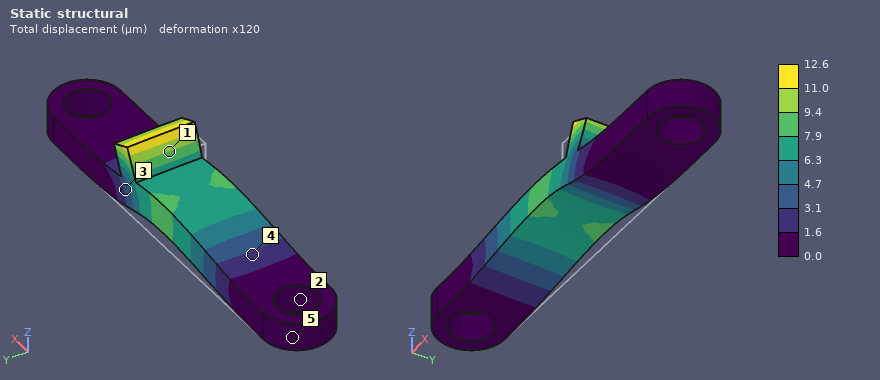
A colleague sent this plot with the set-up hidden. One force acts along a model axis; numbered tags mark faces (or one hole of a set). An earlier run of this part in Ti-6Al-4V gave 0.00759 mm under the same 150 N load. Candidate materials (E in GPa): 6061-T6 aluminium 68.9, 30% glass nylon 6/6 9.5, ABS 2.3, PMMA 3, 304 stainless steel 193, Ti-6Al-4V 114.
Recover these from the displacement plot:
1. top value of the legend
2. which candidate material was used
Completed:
12.6 µm
6061-T6 aluminium
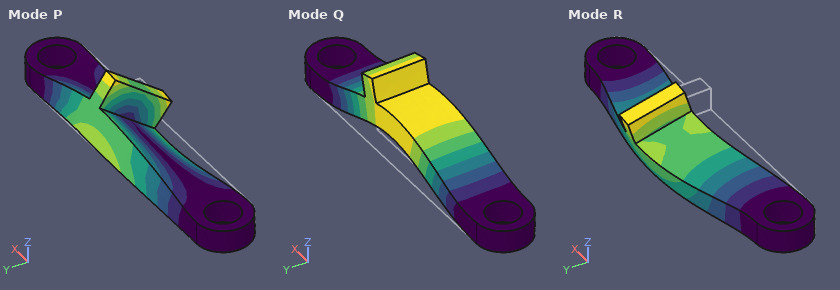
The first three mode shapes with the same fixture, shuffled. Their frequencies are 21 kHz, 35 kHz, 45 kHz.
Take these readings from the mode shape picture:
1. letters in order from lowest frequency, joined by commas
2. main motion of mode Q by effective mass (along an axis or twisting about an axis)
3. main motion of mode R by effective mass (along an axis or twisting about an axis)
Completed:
Q, R, P
along Z
along Y
